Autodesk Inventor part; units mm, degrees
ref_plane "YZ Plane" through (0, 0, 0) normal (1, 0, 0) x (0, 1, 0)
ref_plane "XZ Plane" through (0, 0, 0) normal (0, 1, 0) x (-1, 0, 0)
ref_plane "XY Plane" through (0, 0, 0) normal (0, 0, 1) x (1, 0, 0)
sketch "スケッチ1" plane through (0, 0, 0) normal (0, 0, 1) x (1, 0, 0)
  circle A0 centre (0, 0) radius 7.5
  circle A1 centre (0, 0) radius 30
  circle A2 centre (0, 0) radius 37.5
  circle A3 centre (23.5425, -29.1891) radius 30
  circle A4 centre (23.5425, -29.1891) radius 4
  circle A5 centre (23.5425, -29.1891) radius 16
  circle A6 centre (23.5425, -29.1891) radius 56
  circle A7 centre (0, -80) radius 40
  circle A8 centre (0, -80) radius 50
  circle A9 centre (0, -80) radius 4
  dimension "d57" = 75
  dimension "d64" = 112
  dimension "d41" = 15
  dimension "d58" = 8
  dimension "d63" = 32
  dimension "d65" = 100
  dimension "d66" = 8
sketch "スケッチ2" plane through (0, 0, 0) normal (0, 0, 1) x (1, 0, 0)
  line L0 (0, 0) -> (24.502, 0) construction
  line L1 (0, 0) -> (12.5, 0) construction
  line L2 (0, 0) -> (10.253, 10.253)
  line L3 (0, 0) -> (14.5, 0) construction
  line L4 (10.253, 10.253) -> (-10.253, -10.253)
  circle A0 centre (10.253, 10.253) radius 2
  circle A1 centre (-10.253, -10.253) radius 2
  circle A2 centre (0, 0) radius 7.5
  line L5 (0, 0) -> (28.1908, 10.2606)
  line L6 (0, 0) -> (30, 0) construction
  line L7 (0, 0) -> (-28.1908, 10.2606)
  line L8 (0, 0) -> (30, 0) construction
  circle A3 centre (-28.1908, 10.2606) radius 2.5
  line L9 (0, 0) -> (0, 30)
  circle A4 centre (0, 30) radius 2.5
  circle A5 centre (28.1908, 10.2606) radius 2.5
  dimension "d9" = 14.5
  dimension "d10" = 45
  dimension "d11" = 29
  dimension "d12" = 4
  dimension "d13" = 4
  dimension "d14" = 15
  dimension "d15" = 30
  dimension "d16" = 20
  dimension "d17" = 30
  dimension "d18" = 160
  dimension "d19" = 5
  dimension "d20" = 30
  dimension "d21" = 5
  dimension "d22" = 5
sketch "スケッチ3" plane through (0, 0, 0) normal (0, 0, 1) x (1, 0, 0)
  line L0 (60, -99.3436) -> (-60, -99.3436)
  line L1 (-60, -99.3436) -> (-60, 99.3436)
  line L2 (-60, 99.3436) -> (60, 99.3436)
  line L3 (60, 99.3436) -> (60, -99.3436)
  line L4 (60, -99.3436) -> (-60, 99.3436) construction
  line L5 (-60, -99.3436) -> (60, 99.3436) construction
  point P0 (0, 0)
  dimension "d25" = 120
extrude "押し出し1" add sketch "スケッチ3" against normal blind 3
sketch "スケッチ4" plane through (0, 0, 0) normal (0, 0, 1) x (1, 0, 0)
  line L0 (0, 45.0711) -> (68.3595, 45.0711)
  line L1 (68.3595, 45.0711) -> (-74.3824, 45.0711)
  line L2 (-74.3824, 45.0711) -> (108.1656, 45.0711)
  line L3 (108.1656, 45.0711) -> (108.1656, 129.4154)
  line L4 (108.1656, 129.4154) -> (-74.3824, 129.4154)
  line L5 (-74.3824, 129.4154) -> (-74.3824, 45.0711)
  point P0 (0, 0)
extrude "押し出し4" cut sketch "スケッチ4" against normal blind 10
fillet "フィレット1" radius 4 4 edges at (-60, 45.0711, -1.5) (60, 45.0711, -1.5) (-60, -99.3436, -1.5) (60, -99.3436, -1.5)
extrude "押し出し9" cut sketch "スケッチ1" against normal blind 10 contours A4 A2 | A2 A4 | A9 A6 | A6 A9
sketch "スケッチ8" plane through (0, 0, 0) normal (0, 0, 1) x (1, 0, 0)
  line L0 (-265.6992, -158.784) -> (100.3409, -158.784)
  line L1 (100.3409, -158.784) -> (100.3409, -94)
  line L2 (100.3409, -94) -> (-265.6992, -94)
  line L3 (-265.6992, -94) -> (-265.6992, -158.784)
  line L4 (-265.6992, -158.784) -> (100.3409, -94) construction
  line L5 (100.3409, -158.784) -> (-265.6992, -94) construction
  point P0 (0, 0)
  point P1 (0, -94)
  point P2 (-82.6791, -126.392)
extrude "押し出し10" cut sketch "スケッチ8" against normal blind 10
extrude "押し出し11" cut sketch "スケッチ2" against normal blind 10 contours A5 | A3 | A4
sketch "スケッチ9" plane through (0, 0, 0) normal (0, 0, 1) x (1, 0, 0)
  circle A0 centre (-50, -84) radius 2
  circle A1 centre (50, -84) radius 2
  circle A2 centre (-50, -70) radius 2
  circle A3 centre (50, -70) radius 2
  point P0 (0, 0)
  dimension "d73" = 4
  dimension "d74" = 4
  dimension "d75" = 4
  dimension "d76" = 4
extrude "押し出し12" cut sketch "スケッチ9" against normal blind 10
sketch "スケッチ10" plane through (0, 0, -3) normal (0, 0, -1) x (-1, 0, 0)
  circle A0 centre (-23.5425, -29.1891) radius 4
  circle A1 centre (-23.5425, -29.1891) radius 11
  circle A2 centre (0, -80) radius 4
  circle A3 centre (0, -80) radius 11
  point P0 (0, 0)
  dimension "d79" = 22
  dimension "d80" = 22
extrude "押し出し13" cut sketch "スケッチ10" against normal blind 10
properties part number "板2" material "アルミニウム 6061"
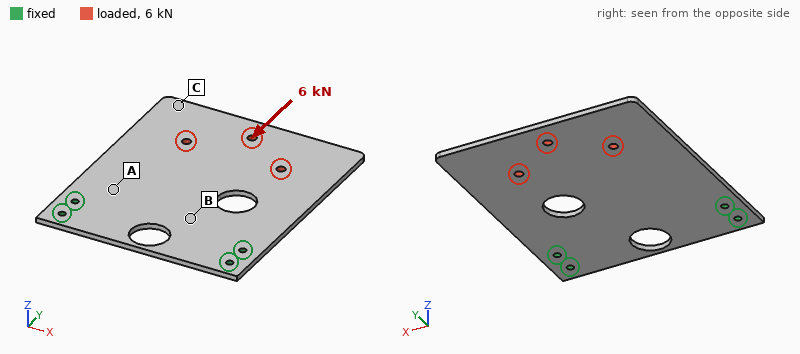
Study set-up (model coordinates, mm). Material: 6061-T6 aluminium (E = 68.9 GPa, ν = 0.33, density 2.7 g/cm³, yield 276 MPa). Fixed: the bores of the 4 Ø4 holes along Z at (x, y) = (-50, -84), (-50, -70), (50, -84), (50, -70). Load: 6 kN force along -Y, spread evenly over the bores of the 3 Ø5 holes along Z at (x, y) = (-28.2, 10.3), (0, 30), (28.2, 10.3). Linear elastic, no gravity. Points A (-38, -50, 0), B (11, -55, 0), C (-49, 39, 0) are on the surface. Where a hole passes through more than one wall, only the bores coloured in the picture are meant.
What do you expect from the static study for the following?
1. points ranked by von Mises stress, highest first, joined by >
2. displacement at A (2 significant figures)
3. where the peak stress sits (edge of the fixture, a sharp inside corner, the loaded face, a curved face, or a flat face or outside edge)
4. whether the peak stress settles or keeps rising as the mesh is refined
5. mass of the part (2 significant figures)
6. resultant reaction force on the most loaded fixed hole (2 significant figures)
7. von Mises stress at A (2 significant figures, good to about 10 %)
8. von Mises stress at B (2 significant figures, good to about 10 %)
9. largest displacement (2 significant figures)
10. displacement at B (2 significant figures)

A > B > C
14 µm
edge of the fixture
keeps rising
130 g
2.1 kN
25 MPa
14 MPa
46 µm
20 µm
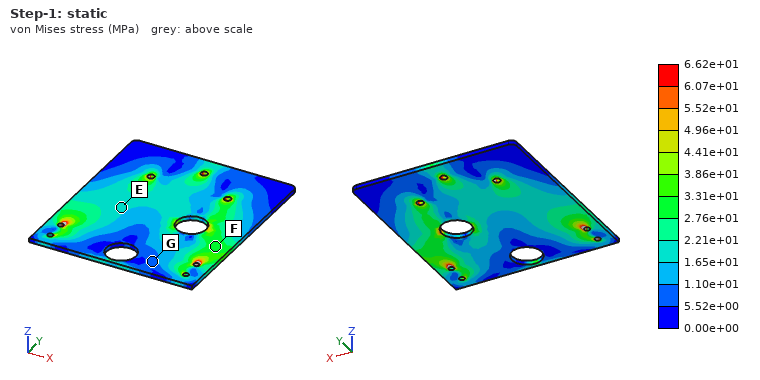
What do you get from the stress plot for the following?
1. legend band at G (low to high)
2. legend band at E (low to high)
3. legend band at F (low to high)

5.52e+00 to 1.10e+01 MPa
1.65e+01 to 2.21e+01 MPa
2.76e+01 to 3.31e+01 MPa
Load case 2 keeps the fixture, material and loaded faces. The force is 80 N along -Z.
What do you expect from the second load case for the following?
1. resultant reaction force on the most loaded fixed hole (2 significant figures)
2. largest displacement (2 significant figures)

160 N
1.9 mm
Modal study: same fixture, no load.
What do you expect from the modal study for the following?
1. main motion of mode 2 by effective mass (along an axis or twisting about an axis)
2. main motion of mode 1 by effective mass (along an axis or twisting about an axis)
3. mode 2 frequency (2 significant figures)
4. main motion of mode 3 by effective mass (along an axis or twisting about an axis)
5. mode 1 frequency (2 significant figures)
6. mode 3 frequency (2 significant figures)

twisting about Y
along Z
430 Hz
along Z
160 Hz
1000 Hz
